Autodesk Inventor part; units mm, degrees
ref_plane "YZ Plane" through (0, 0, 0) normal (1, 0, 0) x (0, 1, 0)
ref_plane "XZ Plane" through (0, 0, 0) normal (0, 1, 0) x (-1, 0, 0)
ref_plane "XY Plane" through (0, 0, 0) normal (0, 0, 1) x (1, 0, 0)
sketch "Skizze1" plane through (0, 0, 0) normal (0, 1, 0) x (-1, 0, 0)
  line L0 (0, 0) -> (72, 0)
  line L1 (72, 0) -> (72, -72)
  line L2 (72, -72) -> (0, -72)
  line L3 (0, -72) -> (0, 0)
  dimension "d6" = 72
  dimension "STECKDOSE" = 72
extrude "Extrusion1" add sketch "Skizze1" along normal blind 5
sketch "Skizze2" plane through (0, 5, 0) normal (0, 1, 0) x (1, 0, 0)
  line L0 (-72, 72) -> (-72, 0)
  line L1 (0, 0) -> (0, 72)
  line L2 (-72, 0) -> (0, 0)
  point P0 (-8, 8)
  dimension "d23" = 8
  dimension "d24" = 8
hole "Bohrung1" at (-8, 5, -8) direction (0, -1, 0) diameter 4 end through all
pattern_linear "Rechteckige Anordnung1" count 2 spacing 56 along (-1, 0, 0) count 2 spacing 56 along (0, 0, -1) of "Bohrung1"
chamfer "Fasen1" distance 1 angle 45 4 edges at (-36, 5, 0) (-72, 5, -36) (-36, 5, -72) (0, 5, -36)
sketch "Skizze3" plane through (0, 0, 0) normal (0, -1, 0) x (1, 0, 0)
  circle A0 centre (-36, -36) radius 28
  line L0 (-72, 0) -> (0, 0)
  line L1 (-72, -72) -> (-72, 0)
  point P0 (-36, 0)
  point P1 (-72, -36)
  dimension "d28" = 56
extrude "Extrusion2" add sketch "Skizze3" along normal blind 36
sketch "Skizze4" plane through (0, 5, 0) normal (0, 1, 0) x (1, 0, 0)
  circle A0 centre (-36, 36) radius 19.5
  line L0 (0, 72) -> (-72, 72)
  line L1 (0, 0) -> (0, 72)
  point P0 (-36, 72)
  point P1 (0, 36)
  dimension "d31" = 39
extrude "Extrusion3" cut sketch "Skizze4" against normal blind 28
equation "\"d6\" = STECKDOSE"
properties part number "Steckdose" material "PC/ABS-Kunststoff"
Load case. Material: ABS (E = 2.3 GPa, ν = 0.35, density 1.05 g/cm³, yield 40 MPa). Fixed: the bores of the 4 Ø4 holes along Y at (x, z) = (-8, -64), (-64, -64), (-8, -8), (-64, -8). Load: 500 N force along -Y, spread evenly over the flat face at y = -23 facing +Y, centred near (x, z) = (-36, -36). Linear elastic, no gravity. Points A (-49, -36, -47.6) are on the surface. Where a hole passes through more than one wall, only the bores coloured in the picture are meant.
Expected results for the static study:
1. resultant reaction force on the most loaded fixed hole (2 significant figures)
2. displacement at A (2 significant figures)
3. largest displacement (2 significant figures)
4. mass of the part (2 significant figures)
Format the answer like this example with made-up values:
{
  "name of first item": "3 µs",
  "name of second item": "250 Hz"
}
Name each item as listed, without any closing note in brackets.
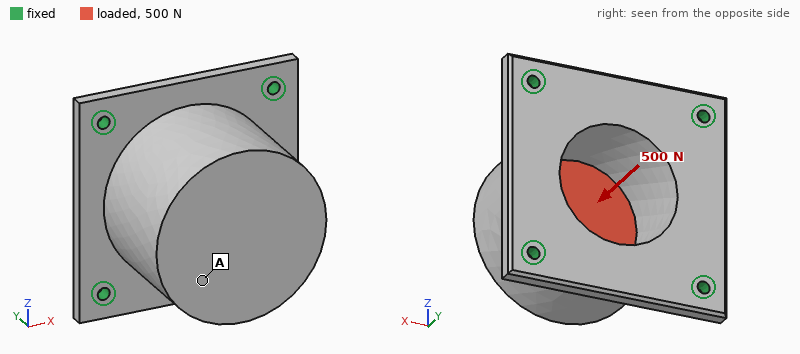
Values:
{
  "resultant reaction force on the most loaded fixed hole": "140 N",
  "displacement at A": "0.095 mm",
  "largest displacement": "0.10 mm",
  "mass of the part": "85 g"
}
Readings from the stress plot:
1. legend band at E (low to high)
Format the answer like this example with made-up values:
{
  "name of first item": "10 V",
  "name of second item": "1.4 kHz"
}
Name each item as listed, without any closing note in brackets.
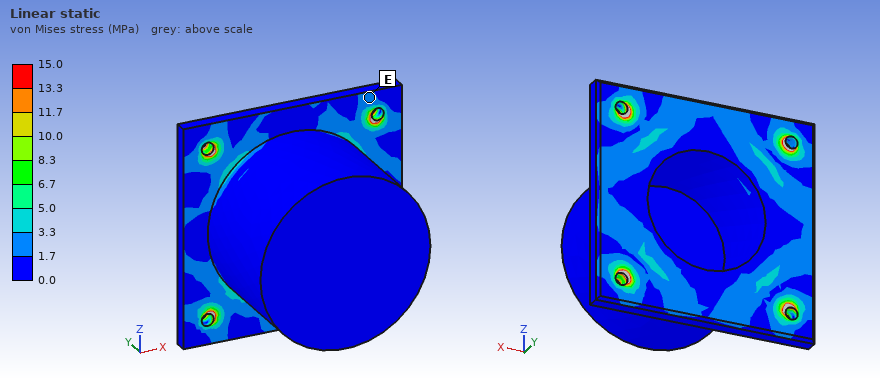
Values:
{
  "legend band at E": "1.7 to 3.3 MPa"
}
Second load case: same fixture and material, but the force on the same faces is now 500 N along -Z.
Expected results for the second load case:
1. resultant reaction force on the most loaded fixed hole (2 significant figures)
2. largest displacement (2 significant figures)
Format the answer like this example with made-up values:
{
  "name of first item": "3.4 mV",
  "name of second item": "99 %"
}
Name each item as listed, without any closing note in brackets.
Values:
{
  "resultant reaction force on the most loaded fixed hole": "180 N",
  "largest displacement": "0.20 mm"
}
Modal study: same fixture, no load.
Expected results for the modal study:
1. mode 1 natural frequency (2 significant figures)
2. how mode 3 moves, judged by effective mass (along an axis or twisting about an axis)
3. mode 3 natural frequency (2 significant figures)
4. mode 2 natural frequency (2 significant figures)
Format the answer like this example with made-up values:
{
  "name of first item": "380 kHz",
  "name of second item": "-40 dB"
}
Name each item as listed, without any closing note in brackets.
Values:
{
  "mode 1 natural frequency": "1100 Hz",
  "how mode 3 moves, judged by effective mass": "along Y",
  "mode 3 natural frequency": "1300 Hz",
  "mode 2 natural frequency": "1100 Hz"
}
